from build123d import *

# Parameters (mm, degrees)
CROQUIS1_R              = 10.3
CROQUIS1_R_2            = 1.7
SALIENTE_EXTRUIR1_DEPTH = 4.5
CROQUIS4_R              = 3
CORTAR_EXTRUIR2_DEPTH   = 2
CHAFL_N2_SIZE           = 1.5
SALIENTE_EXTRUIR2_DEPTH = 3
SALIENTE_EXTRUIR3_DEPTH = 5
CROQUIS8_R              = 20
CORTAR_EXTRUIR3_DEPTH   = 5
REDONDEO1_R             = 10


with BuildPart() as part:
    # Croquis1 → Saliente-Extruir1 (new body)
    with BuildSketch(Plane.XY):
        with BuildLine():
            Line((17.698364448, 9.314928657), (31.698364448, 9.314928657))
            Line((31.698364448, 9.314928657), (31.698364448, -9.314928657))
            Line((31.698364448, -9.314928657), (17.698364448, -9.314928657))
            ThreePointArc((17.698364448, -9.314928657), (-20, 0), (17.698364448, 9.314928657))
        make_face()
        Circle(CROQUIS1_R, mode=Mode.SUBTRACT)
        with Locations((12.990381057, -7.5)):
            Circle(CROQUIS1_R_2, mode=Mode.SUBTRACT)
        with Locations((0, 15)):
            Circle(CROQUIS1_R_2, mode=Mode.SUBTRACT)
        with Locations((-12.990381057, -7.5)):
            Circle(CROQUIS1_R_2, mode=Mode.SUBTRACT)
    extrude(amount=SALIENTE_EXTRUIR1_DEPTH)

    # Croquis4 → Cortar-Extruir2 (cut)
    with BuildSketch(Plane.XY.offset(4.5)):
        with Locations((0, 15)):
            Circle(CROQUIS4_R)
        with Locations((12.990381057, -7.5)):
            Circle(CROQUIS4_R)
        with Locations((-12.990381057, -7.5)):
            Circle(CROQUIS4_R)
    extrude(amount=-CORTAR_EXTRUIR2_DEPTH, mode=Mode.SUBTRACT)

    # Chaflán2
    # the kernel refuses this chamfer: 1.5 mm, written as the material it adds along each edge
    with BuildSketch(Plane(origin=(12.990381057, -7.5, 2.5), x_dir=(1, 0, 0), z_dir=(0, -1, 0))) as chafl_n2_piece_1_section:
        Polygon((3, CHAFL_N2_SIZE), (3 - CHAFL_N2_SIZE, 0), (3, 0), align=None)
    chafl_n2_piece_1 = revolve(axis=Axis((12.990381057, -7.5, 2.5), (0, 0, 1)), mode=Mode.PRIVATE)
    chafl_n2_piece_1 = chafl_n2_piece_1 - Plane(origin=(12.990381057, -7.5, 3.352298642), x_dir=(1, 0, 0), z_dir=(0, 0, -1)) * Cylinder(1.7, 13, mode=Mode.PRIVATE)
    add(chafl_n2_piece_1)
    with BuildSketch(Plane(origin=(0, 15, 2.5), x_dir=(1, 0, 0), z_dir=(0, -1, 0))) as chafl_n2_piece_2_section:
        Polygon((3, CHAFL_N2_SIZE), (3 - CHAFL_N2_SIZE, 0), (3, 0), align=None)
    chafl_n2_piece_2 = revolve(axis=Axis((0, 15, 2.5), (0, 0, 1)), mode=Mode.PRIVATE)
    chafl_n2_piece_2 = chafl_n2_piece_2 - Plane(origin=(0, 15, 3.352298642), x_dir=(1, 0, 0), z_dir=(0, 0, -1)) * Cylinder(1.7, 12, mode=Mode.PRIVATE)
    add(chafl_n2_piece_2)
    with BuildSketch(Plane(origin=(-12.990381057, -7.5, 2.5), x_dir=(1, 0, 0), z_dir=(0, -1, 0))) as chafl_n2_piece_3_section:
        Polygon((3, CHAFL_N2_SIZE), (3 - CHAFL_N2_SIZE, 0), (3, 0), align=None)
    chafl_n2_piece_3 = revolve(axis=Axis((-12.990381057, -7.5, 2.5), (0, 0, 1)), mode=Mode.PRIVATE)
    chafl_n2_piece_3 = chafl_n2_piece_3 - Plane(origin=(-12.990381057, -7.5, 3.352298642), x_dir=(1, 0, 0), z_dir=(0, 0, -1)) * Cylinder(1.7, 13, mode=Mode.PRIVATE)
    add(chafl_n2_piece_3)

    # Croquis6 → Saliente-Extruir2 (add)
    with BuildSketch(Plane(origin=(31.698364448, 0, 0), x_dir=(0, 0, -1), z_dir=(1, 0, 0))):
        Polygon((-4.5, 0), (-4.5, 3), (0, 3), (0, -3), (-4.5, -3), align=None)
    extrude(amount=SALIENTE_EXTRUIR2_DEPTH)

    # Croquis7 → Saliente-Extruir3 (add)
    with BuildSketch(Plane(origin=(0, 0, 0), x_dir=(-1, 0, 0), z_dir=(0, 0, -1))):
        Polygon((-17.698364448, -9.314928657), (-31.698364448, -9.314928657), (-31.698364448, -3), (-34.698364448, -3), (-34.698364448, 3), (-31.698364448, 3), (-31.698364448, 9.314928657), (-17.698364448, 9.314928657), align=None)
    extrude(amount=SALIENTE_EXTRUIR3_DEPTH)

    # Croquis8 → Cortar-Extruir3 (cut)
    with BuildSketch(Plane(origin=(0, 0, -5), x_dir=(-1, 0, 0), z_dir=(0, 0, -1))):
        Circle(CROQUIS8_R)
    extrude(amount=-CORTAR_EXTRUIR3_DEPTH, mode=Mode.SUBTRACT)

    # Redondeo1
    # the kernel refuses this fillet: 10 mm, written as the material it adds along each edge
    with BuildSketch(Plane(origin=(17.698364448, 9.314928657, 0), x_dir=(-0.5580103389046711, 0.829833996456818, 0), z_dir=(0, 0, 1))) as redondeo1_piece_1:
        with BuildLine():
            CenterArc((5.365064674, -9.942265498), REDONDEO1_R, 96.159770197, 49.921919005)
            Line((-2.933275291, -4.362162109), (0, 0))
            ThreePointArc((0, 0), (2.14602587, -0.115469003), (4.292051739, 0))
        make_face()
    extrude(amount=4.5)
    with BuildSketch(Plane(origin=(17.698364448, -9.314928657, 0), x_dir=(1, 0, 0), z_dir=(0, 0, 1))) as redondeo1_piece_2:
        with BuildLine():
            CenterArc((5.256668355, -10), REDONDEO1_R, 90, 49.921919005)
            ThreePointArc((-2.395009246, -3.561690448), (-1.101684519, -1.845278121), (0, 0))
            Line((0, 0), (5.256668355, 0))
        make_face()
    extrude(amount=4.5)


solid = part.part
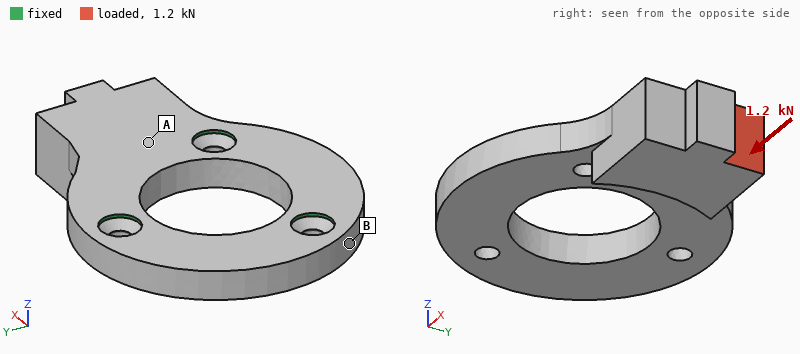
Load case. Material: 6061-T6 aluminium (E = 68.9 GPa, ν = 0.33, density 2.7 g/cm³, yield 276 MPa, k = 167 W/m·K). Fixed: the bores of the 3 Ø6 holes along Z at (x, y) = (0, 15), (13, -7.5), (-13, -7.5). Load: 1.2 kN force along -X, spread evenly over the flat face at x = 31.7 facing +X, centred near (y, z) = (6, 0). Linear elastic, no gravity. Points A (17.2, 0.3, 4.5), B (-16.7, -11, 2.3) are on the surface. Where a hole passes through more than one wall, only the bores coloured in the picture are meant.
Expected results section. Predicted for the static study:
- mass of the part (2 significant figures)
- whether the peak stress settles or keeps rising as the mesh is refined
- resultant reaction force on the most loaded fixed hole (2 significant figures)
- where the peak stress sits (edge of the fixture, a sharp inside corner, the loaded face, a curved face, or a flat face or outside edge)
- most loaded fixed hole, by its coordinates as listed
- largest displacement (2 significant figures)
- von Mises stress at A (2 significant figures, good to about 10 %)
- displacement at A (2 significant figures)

17 g
keeps rising
830 N
edge of the fixture
(0, 15)
85 µm
23 MPa
13 µm
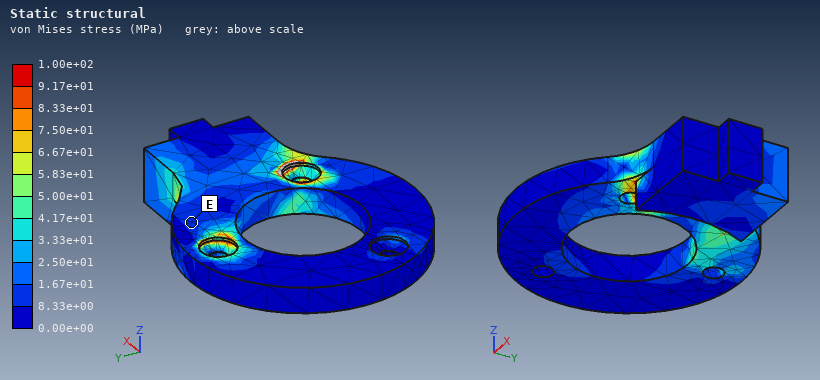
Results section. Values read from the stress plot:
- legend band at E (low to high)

8.33e+00 to 1.67e+01 MPa
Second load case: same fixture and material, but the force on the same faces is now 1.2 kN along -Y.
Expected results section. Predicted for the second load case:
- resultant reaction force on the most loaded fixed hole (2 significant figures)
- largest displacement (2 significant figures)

1.2 kN
52 µm
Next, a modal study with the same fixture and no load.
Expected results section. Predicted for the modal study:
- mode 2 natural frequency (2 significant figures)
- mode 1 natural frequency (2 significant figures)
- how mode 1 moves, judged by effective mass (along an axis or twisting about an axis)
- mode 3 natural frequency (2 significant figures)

13 kHz
4600 Hz
along Z
15 kHz
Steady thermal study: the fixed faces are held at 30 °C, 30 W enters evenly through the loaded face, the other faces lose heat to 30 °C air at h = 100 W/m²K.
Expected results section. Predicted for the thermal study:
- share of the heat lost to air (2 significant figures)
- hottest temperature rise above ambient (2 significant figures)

12 %
44 K
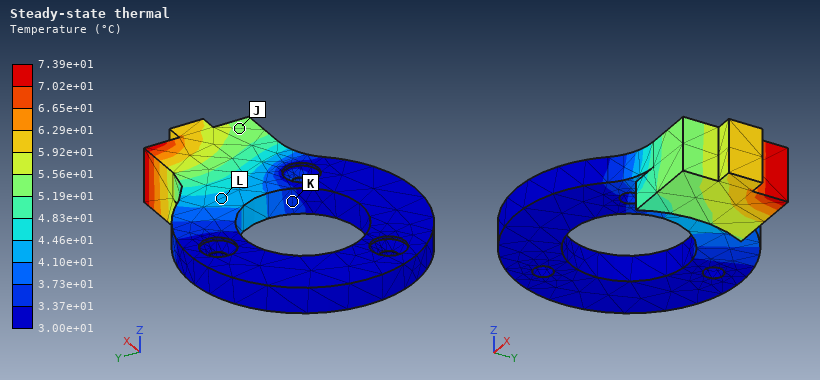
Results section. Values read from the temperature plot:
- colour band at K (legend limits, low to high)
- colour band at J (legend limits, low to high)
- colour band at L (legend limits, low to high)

3.37e+01 to 3.73e+01 °C
5.19e+01 to 5.56e+01 °C
4.10e+01 to 4.46e+01 °C
